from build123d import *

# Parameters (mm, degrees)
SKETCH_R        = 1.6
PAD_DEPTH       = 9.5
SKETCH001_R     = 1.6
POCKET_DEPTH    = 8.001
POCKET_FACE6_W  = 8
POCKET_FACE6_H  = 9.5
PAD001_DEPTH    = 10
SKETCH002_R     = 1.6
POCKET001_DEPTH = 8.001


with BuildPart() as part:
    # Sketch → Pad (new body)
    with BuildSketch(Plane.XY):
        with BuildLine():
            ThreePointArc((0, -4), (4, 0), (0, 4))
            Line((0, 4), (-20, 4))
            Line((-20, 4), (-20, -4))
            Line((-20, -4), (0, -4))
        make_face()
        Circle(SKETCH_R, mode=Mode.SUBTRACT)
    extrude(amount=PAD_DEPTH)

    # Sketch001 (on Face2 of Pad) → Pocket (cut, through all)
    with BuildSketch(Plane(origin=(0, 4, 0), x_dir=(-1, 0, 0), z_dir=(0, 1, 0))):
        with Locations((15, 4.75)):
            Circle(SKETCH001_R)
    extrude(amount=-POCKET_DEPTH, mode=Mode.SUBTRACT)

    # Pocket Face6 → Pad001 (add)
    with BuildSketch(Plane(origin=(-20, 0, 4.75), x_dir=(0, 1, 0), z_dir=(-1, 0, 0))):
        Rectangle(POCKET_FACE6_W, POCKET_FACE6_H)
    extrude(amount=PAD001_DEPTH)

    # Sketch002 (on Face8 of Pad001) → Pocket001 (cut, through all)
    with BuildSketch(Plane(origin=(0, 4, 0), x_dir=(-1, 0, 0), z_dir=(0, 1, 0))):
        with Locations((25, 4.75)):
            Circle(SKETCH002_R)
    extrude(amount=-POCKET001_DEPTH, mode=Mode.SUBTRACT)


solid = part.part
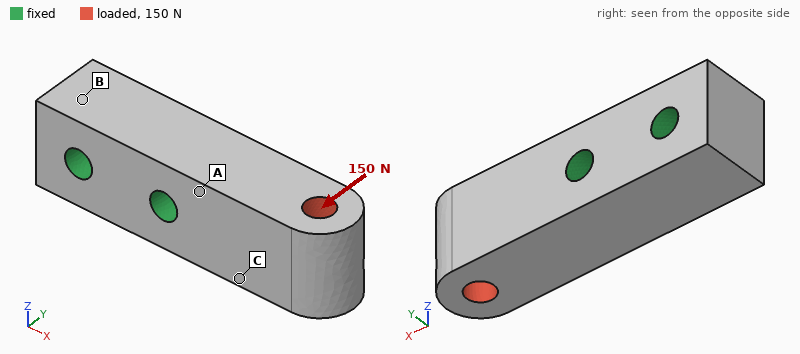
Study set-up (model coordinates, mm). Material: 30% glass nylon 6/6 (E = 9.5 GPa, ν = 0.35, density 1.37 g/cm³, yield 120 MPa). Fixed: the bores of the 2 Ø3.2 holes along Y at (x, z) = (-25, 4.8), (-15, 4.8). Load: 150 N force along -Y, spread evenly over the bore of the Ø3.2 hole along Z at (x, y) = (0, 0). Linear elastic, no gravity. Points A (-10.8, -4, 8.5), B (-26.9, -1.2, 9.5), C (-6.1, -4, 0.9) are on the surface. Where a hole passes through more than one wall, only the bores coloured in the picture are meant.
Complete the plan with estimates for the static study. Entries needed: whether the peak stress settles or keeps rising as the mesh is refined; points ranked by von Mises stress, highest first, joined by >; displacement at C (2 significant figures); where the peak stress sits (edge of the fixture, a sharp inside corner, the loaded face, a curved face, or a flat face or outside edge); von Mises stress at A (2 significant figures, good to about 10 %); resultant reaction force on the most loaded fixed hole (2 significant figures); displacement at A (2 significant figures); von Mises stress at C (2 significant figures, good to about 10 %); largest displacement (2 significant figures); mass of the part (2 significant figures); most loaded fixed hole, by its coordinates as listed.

keeps rising
A > C > B
27 µm
edge of the fixture
14 MPa
180 N
11 µm
9.0 MPa
70 µm
3.2 g
(-15, 4.8)
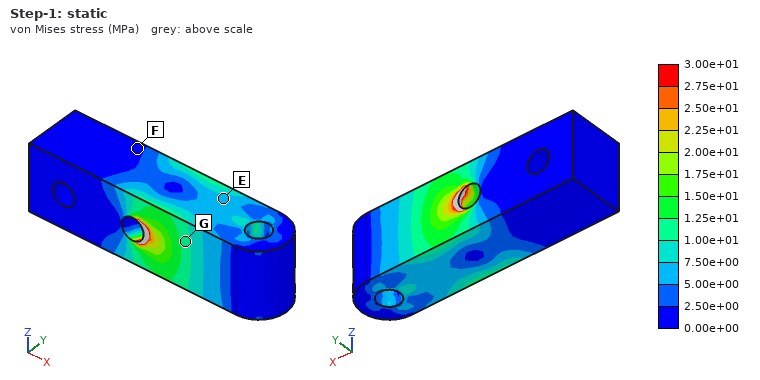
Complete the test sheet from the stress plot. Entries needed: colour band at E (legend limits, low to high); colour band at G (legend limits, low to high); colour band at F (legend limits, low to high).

5.00e+00 to 7.50e+00 MPa
1.00e+01 to 1.25e+01 MPa
0.00e+00 to 2.50e+00 MPa
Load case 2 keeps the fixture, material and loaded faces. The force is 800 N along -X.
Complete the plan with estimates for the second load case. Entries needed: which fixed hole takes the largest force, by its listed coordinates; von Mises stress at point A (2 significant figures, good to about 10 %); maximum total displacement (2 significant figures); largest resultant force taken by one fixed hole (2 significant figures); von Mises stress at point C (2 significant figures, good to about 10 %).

(-15, 4.8)
8.3 MPa
24 µm
720 N
11 MPa
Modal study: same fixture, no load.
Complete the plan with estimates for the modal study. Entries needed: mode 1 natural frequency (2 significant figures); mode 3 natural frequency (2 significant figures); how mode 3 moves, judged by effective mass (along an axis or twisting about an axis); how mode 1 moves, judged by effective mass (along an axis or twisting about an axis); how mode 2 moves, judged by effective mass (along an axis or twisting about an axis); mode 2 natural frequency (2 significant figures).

9400 Hz
21 kHz
twisting about X
along Z
along Y
9800 Hz
